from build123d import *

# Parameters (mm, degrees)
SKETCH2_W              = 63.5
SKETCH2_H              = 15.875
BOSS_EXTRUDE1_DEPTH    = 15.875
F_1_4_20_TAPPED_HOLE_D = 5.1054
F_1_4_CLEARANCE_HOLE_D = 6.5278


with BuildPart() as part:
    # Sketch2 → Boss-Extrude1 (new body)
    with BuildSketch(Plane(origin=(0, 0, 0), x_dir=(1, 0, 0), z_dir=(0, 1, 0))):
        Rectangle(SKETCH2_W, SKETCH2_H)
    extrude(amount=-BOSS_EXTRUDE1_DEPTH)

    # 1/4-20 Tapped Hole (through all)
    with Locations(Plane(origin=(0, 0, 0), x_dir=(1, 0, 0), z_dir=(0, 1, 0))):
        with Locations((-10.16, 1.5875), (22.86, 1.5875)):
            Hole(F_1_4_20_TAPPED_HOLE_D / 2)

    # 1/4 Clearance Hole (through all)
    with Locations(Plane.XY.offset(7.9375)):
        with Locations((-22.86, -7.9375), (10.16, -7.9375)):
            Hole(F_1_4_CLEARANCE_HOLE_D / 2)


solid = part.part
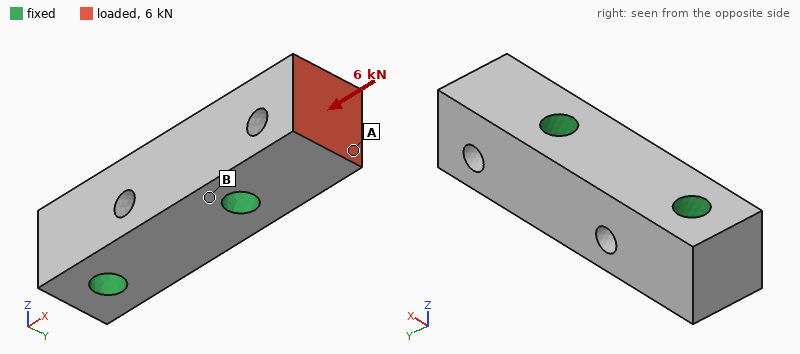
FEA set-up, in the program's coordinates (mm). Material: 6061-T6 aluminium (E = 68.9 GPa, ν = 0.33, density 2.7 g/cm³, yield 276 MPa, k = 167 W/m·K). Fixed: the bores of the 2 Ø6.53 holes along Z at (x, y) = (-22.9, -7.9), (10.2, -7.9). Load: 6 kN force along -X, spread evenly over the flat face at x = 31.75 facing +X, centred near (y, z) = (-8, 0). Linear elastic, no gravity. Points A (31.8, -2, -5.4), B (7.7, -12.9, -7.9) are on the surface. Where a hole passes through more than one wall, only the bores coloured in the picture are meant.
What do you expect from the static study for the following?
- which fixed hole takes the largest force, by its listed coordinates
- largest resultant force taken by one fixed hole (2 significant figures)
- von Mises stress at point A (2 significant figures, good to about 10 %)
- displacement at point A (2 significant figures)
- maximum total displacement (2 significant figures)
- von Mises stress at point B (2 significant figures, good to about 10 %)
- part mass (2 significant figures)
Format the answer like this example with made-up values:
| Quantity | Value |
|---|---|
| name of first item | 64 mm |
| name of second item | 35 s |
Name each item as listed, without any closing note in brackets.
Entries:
| Quantity | Value |
|---|---|
| which fixed hole takes the largest force, by its listed coordinates | (10.2, -7.9) |
| largest resultant force taken by one fixed hole | 5.8 kN |
| von Mises stress at point A | 22 MPa |
| displacement at point A | 9.3 µm |
| maximum total displacement | 9.8 µm |
| von Mises stress at point B | 8.5 MPa |
| part mass | 39 g |
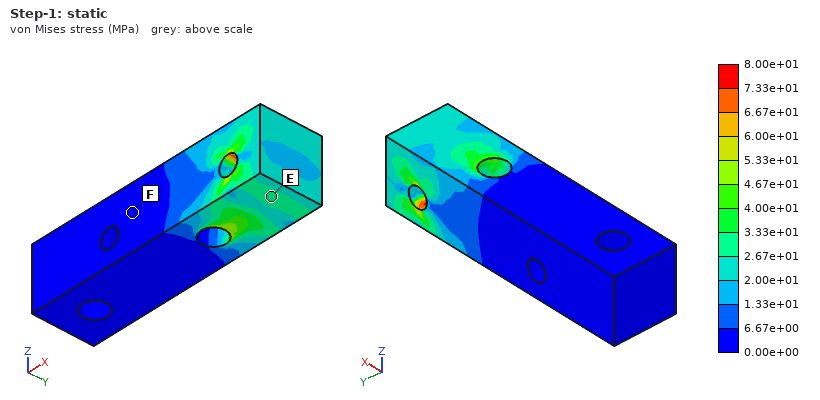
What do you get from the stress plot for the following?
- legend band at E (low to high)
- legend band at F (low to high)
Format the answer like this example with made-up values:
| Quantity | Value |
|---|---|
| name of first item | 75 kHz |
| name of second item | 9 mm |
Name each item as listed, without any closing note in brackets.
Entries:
| Quantity | Value |
|---|---|
| legend band at E | 2.67e+01 to 3.33e+01 MPa |
| legend band at F | 0.00e+00 to 6.67e+00 MPa |
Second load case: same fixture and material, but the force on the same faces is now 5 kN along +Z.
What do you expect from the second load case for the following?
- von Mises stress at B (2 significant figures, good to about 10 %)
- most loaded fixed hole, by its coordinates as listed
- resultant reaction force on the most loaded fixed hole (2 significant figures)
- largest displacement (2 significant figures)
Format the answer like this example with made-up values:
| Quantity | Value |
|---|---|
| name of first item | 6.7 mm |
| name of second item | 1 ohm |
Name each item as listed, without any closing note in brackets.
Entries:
| Quantity | Value |
|---|---|
| von Mises stress at B | 35 MPa |
| most loaded fixed hole, by its coordinates as listed | (10.2, -7.9) |
| resultant reaction force on the most loaded fixed hole | 5.2 kN |
| largest displacement | 72 µm |
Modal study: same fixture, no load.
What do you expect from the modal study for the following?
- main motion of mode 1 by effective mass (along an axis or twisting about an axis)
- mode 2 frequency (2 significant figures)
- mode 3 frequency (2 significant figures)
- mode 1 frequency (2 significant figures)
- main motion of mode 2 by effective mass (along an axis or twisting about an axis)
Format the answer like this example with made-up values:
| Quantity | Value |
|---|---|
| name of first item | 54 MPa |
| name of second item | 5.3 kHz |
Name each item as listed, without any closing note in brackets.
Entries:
| Quantity | Value |
|---|---|
| main motion of mode 1 by effective mass | along Y |
| mode 2 frequency | 22 kHz |
| mode 3 frequency | 34 kHz |
| mode 1 frequency | 19 kHz |
| main motion of mode 2 by effective mass | along Z |
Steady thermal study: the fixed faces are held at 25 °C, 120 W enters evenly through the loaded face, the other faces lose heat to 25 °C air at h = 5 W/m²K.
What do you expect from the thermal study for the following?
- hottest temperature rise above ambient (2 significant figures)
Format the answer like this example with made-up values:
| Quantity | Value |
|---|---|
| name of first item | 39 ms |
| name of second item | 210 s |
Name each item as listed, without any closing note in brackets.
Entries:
| Quantity | Value |
|---|---|
| hottest temperature rise above ambient | 66 K |
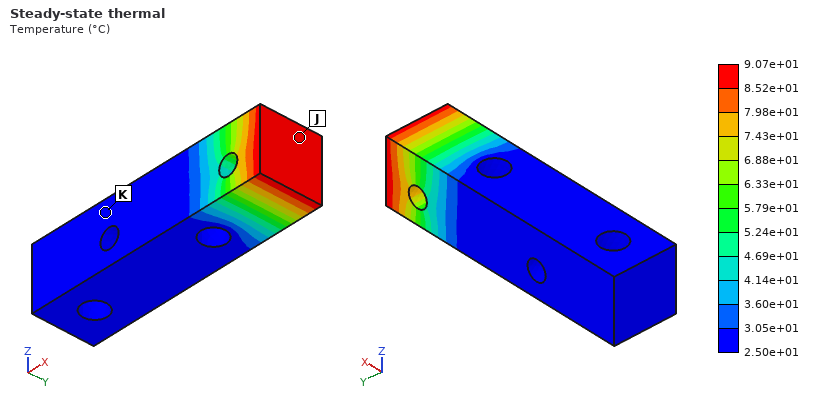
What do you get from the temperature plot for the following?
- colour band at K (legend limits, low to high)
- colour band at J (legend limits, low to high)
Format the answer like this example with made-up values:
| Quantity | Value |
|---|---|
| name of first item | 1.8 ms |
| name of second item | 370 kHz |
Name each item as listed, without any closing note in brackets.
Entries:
| Quantity | Value |
|---|---|
| colour band at K | 2.50e+01 to 3.05e+01 °C |
| colour band at J | 8.52e+01 to 9.07e+01 °C |
